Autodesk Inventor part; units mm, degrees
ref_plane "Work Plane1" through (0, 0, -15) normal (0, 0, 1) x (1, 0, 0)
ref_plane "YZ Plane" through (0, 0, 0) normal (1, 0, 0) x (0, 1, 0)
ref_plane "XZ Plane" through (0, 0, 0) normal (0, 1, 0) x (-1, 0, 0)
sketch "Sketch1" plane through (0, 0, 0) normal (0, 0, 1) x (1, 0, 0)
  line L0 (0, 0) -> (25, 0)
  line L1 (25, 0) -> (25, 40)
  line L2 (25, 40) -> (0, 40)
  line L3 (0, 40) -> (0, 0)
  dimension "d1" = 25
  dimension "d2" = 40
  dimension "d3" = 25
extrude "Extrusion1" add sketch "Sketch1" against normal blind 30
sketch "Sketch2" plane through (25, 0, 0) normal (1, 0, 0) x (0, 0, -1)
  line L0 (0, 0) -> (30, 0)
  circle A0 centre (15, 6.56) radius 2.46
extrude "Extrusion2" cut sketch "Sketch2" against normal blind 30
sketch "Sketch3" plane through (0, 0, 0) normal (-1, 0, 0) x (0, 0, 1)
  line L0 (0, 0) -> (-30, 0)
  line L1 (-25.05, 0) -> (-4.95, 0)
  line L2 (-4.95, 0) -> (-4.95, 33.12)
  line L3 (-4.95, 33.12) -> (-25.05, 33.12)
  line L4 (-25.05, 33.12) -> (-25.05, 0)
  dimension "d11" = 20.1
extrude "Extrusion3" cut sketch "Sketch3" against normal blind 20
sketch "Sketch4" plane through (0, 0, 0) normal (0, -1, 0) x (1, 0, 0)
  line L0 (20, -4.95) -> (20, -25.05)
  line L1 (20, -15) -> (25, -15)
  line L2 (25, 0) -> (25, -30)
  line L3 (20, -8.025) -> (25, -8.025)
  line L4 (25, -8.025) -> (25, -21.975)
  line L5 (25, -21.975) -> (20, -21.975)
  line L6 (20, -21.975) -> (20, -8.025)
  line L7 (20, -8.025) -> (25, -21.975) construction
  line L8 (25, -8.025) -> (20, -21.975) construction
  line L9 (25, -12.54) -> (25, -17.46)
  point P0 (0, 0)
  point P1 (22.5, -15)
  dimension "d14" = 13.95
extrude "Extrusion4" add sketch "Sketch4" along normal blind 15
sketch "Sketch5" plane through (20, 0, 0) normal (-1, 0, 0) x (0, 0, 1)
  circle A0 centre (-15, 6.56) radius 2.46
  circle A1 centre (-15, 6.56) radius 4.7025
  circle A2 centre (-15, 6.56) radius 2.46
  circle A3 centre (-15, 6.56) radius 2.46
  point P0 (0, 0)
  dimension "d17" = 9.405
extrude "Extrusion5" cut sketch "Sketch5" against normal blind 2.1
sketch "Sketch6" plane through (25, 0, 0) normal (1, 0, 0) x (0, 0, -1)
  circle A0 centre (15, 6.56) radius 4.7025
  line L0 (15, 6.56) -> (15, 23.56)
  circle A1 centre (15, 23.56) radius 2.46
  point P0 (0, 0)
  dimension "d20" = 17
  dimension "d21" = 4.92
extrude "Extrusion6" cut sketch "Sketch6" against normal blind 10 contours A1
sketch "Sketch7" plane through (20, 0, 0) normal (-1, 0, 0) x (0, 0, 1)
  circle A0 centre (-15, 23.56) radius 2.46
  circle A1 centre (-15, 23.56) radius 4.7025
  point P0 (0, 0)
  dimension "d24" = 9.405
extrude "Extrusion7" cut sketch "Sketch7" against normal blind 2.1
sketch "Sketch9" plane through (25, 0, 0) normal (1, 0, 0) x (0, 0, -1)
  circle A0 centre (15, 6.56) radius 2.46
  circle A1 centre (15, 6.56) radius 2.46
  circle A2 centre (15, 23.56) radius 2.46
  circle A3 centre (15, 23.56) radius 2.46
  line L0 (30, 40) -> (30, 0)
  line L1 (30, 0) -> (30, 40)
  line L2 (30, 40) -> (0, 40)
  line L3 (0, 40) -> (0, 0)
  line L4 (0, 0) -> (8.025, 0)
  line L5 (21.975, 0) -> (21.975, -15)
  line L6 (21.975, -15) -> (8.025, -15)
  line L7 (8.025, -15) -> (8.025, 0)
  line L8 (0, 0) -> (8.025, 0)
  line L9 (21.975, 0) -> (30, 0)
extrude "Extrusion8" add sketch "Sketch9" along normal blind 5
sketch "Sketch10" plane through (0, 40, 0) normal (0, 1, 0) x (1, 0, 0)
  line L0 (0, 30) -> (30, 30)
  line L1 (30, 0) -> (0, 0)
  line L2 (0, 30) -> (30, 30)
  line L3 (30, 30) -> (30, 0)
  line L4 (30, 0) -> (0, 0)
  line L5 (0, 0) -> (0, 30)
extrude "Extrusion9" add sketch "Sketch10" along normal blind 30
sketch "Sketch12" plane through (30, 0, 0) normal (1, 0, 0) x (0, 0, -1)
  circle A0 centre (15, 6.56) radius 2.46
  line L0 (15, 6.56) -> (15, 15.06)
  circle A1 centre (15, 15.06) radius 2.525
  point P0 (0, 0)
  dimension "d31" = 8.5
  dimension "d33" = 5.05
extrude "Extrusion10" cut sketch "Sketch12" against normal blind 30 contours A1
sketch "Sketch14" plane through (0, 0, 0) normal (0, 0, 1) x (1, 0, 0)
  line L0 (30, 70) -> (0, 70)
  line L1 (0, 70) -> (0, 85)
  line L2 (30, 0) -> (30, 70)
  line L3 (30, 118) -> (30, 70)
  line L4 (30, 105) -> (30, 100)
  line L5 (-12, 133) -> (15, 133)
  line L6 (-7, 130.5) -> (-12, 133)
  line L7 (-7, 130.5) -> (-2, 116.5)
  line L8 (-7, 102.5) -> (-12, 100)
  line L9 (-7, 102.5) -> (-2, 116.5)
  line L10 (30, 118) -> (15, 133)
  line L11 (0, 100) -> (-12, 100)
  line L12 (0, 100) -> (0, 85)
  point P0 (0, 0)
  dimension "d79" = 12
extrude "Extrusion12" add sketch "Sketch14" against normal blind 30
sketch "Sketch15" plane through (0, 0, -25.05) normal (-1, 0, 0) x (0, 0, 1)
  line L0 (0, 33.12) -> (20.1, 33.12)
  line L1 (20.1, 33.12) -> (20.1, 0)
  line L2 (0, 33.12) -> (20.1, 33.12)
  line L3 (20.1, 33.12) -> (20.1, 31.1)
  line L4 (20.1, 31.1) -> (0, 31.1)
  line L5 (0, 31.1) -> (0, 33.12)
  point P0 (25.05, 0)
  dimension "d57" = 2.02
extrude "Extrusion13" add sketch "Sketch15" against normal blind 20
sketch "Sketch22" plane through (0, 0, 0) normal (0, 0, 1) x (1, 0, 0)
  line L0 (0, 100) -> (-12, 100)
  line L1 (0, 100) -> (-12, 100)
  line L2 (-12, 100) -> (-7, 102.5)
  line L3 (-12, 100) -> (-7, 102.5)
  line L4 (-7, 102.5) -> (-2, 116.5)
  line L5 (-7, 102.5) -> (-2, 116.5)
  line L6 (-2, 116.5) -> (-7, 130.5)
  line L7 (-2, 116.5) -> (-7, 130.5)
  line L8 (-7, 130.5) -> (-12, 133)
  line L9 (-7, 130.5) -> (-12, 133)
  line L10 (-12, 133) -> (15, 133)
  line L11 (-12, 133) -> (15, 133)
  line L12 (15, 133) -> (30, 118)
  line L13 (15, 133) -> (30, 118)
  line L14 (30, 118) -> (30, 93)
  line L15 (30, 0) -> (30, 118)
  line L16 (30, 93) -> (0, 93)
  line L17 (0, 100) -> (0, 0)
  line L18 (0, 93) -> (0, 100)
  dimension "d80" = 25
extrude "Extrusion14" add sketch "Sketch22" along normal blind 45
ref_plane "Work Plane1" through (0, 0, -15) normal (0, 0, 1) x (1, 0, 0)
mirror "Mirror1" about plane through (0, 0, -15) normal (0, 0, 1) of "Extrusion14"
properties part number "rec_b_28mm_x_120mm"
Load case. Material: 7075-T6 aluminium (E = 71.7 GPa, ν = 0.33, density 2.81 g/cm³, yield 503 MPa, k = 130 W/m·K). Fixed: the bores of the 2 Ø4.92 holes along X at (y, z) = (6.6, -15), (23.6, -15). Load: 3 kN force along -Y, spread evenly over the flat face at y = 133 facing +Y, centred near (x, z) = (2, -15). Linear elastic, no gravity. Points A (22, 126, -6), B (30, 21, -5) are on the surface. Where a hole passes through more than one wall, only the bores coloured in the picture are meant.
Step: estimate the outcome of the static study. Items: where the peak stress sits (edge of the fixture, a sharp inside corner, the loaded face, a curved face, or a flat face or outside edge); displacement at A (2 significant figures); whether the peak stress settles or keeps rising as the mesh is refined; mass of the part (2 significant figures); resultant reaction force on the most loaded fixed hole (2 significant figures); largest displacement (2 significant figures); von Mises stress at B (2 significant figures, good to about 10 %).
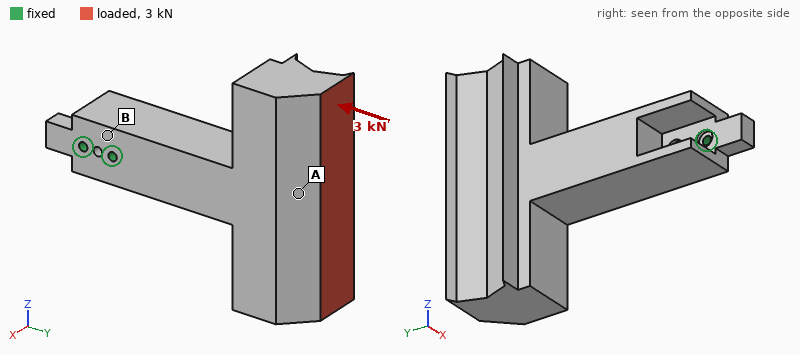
edge of the fixture
0.19 mm
keeps rising
630 g
3.4 kN
0.22 mm
19 MPa
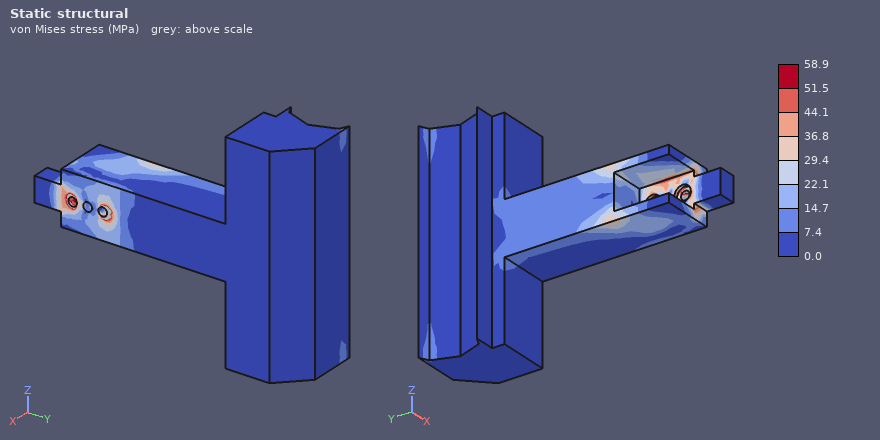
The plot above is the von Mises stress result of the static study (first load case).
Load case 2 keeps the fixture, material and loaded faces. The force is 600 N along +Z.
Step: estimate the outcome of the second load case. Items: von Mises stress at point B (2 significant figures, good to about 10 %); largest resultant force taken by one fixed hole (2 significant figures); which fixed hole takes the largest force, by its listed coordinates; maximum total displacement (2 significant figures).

22 MPa
3.4 kN
(23.6, -15)
0.19 mm
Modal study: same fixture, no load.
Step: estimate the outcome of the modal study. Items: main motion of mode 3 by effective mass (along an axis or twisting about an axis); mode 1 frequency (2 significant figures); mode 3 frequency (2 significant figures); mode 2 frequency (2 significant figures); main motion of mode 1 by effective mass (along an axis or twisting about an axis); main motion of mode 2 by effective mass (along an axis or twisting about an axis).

twisting about Y
500 Hz
810 Hz
540 Hz
along X
along Z
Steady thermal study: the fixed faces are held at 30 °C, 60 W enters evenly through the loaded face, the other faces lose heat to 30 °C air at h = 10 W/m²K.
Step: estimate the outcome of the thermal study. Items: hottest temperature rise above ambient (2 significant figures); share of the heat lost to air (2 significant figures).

54 K
19 %
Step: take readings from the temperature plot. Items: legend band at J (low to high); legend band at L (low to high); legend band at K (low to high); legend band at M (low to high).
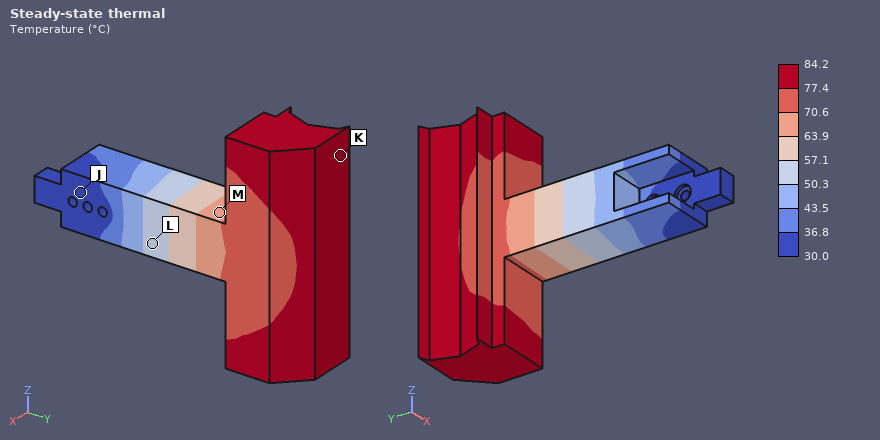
30.0 to 36.8 °C
50.3 to 57.1 °C
77.4 to 84.2 °C
63.9 to 70.6 °C
